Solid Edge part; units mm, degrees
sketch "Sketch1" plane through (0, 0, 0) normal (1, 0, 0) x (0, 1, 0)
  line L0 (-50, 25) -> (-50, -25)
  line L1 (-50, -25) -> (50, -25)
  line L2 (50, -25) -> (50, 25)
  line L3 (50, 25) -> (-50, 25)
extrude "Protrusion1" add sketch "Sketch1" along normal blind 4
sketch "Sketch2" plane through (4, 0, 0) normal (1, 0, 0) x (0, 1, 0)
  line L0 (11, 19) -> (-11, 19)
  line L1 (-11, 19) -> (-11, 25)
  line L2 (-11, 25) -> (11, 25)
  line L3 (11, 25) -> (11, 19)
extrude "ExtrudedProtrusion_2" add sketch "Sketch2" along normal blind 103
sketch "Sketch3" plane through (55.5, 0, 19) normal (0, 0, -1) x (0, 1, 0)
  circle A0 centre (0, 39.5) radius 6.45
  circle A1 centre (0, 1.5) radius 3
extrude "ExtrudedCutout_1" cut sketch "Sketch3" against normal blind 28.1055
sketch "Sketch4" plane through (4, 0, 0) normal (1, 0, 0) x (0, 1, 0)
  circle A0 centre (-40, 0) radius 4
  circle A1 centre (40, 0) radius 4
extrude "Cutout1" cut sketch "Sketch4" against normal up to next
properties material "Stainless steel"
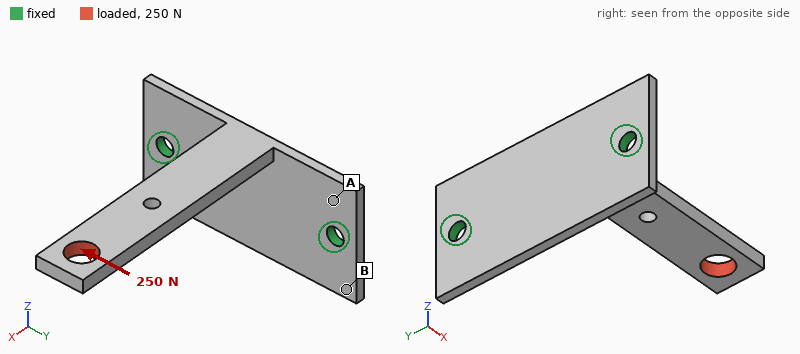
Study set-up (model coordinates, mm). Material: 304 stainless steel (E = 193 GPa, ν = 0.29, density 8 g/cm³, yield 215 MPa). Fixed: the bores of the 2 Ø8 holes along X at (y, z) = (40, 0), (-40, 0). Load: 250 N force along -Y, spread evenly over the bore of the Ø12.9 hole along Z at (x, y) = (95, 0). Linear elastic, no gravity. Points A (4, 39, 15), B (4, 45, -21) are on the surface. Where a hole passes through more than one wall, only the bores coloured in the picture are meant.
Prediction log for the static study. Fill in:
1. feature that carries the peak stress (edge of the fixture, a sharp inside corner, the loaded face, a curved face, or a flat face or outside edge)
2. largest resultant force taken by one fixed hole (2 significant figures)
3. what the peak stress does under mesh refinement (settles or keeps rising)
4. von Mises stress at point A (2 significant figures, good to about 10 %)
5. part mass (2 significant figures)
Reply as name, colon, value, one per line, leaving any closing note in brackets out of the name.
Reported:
feature that carries the peak stress: a sharp inside corner
largest resultant force taken by one fixed hole: 440 N
what the peak stress does under mesh refinement: keeps rising
von Mises stress at point A: 29 MPa
part mass: 260 g
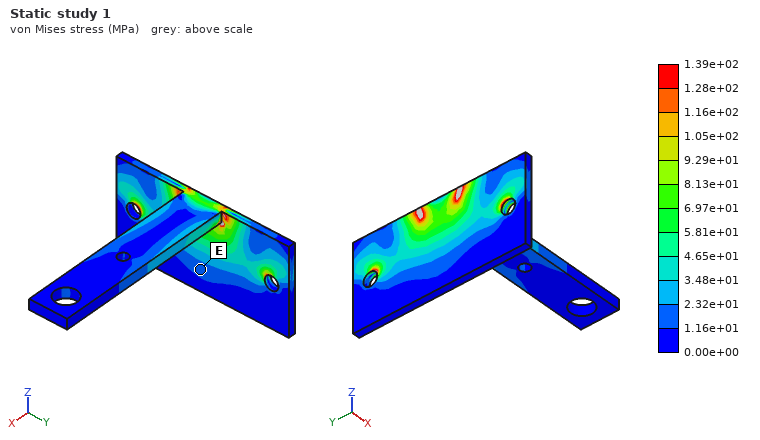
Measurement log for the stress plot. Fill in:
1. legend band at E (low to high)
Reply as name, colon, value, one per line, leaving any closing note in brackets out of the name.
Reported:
legend band at E: 1.16e+01 to 2.32e+01 MPa
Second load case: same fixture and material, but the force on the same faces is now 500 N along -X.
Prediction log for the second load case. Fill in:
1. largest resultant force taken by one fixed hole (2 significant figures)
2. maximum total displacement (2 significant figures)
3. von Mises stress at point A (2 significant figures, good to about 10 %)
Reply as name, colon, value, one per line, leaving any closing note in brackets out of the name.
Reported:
largest resultant force taken by one fixed hole: 260 N
maximum total displacement: 0.27 mm
von Mises stress at point A: 35 MPa
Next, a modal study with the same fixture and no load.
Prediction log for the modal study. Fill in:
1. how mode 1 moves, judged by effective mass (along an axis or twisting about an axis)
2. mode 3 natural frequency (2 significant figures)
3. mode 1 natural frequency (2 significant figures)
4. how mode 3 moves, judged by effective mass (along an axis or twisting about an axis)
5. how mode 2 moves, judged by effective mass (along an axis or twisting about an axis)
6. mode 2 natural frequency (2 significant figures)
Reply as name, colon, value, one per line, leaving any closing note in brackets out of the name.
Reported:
how mode 1 moves, judged by effective mass: along Z
mode 3 natural frequency: 1400 Hz
mode 1 natural frequency: 310 Hz
how mode 3 moves, judged by effective mass: along X
how mode 2 moves, judged by effective mass: along Y
mode 2 natural frequency: 650 Hz
